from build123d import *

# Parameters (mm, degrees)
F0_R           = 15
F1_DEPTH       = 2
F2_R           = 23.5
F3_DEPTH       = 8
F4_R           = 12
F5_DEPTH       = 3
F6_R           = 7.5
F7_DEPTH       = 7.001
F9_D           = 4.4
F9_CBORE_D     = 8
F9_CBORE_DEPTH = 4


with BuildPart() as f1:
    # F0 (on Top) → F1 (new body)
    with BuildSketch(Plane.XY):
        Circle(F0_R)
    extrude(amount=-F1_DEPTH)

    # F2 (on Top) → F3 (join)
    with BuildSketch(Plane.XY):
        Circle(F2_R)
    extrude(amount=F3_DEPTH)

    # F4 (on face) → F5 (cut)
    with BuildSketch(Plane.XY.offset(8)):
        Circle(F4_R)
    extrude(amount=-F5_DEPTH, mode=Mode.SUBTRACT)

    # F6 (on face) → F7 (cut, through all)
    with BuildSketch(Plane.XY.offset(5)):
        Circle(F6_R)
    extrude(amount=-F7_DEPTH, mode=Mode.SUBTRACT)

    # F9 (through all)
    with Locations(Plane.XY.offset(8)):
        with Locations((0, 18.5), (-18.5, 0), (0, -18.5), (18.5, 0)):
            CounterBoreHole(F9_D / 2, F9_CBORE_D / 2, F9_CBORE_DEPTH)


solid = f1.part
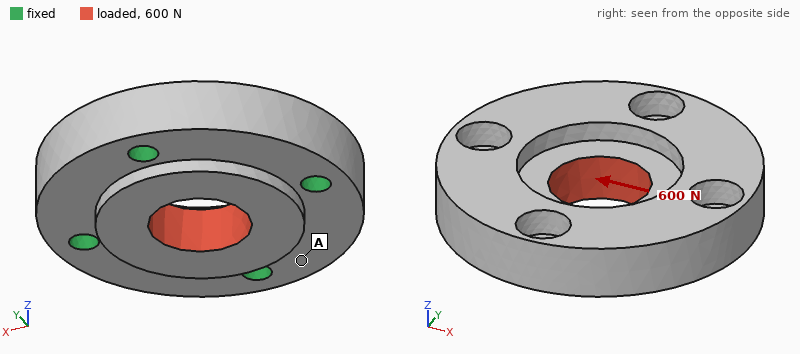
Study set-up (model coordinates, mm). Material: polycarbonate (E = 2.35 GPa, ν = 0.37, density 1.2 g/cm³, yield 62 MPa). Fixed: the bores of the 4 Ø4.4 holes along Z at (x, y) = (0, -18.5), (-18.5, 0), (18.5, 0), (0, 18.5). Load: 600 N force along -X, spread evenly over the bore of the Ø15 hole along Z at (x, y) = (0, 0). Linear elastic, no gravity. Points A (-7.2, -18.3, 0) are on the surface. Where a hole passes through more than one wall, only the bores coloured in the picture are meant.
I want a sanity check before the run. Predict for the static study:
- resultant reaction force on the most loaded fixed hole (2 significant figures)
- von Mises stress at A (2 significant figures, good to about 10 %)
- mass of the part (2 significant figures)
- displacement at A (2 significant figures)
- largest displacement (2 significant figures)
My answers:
180 N
1.4 MPa
14 g
4.1 µm
17 µm
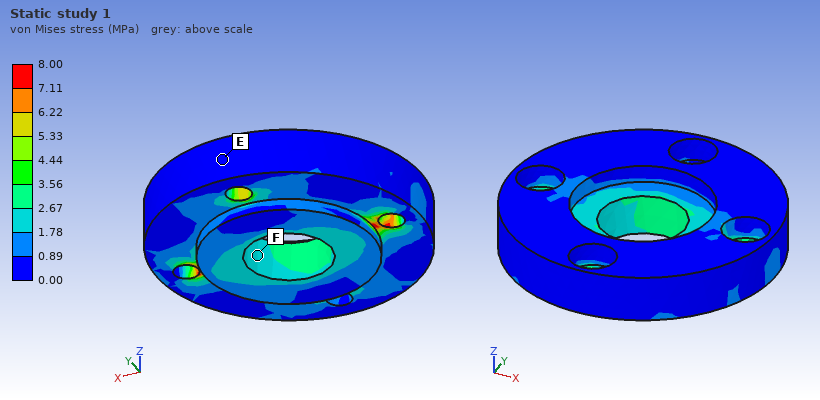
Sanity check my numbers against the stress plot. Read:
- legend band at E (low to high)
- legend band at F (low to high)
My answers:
0.00 to 0.89 MPa
1.78 to 2.67 MPa
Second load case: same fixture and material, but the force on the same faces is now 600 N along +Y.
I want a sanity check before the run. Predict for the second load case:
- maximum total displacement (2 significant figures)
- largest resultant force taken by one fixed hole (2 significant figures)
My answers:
17 µm
180 N
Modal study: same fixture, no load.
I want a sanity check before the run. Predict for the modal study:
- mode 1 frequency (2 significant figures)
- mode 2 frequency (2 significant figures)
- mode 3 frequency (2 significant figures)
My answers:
6200 Hz
7200 Hz
7200 Hz
